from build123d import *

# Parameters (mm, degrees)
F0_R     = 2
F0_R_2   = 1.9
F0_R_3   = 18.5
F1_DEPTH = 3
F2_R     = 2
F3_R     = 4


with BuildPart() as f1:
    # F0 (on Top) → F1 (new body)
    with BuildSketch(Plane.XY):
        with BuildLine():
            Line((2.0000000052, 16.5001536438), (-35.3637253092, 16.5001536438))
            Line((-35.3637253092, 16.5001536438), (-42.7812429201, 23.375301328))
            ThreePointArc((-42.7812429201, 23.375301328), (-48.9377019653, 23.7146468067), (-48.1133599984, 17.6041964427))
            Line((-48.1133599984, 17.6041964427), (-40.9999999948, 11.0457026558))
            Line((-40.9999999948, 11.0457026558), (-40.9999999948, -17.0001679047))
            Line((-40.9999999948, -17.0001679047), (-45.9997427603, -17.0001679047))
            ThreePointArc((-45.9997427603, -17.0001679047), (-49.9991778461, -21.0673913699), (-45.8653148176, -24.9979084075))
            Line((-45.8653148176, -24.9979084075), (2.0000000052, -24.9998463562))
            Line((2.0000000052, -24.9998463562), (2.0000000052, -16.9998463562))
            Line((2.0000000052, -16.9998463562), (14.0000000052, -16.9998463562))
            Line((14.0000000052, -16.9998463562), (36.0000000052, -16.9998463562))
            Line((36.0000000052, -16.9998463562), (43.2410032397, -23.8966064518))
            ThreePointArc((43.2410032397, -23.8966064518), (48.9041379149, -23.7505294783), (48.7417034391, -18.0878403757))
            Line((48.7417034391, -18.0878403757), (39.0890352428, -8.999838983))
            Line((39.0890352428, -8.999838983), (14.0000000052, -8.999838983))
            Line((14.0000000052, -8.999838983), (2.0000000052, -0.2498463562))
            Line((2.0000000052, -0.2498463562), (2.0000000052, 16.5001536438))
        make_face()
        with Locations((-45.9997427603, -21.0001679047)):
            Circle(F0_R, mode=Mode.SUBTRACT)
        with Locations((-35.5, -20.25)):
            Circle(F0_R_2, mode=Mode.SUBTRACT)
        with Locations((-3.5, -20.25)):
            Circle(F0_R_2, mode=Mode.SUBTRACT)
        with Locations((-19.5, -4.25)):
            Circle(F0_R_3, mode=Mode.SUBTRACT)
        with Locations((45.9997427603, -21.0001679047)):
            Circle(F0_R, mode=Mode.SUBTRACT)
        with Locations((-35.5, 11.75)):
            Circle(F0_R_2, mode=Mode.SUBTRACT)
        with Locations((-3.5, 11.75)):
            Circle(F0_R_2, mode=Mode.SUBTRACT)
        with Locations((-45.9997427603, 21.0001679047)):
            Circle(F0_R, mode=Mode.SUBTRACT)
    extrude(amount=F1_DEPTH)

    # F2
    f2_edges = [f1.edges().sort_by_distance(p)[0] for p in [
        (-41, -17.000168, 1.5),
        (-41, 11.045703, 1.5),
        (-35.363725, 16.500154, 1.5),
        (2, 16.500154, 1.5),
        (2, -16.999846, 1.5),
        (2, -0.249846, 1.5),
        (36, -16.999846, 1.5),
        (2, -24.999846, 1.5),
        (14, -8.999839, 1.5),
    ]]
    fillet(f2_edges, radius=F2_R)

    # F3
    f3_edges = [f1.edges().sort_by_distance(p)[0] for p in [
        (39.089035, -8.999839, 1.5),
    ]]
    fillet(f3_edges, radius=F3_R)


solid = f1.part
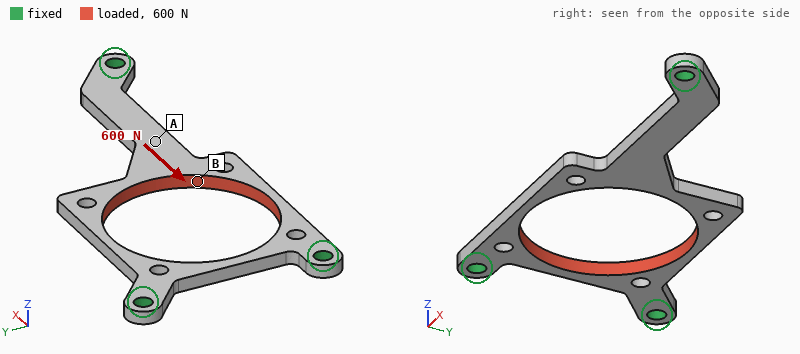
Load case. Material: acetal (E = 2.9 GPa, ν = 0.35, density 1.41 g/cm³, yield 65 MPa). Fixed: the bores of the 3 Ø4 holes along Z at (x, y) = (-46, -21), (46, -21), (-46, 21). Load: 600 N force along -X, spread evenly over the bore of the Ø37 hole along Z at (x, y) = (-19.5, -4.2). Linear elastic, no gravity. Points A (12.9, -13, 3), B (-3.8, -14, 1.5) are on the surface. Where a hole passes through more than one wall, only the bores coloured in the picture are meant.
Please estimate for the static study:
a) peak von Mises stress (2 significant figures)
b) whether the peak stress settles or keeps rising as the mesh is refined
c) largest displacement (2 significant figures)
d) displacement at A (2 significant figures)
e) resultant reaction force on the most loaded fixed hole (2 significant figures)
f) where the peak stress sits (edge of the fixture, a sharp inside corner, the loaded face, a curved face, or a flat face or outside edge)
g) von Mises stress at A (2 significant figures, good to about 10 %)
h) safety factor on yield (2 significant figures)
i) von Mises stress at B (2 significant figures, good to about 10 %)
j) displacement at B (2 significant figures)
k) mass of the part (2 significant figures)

56 MPa
settles
0.67 mm
0.40 mm
260 N
a curved face
4.7 MPa
1.2
13 MPa
0.58 mm
5.2 g
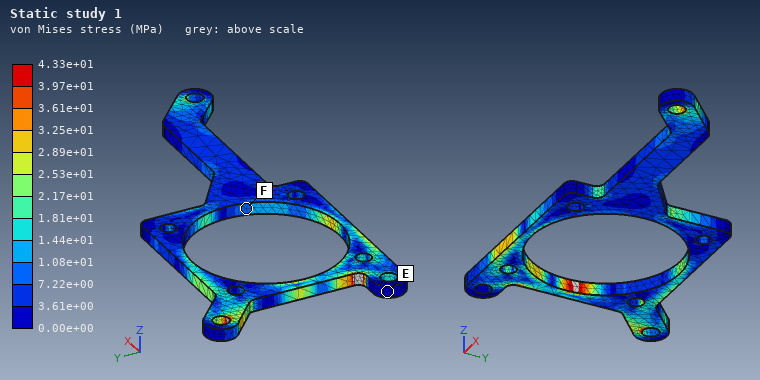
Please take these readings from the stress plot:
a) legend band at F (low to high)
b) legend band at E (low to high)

7.22e+00 to 1.08e+01 MPa
0.00e+00 to 3.61e+00 MPa
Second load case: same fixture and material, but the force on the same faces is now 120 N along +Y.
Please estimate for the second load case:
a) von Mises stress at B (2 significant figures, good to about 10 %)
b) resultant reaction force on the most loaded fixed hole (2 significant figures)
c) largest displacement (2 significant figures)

11 MPa
46 N
0.93 mm
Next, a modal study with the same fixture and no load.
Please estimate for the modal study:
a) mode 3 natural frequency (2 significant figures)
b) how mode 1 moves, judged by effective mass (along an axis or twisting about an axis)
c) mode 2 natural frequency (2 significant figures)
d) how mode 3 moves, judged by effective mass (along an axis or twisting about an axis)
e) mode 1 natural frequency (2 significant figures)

940 Hz
along Z
670 Hz
along Y
410 Hz
